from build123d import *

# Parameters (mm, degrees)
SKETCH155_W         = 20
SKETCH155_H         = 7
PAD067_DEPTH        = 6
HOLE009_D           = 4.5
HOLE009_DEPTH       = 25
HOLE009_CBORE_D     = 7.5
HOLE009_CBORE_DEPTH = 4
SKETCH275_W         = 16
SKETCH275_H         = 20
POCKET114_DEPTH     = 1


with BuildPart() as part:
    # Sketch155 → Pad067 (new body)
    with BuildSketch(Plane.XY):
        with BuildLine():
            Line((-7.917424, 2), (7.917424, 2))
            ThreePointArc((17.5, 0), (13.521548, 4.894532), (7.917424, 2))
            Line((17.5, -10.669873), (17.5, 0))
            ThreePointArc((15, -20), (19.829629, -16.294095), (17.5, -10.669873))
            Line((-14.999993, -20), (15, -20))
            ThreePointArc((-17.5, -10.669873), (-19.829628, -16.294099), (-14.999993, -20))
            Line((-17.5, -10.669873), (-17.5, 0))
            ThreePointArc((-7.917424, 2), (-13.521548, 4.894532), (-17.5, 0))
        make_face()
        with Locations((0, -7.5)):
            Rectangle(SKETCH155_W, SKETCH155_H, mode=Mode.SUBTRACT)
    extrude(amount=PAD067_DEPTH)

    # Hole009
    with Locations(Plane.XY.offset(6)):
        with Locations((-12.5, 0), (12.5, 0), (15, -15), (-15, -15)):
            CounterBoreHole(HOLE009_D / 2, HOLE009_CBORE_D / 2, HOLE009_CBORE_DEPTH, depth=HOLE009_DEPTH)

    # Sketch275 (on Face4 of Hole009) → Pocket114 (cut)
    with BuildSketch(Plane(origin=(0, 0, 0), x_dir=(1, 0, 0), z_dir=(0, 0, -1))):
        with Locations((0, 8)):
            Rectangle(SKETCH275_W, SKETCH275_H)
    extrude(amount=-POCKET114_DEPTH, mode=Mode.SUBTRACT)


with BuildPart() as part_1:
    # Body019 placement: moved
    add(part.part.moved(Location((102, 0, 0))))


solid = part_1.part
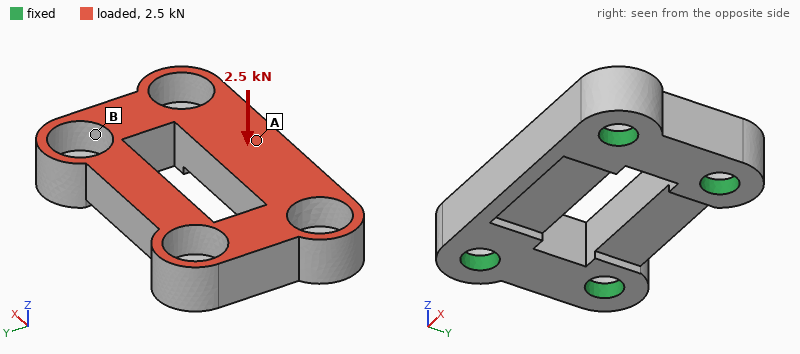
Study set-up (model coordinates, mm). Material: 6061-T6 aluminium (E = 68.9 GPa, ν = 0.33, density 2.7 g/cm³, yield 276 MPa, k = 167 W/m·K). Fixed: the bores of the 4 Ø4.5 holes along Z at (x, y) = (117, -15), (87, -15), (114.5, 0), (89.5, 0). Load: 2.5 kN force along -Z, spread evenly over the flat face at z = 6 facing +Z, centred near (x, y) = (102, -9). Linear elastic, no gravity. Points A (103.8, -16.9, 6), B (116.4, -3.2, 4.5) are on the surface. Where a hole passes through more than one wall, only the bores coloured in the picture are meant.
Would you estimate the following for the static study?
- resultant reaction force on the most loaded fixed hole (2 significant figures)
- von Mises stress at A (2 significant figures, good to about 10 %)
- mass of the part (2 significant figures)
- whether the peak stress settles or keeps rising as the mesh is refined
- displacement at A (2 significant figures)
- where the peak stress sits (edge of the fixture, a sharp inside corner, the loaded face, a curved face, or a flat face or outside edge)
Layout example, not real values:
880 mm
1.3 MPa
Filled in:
920 N
44 MPa
8.5 g
keeps rising
17 µm
edge of the fixture
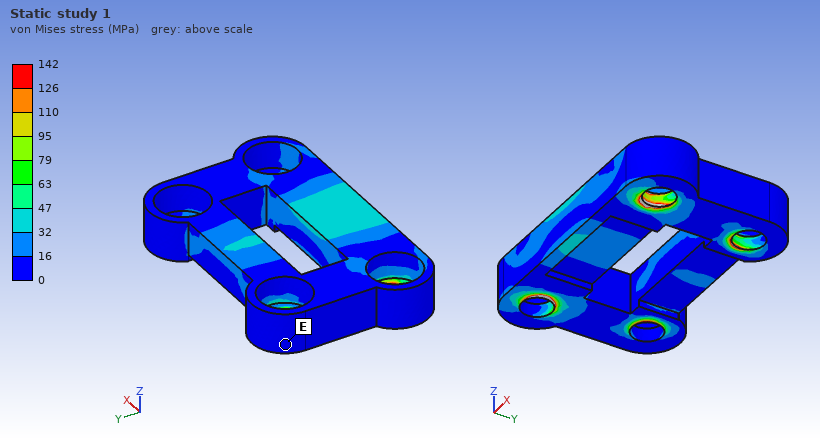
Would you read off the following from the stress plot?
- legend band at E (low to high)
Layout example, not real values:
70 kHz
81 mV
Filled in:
0 to 16 MPa
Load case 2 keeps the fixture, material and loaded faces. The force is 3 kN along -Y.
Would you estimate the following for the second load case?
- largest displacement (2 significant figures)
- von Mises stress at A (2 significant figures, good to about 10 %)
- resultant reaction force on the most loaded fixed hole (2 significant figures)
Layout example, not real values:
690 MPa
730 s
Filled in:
23 µm
16 MPa
900 N
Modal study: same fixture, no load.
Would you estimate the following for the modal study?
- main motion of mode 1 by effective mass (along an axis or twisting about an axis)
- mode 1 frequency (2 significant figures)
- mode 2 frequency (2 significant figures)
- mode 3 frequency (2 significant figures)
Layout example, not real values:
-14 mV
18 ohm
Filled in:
along Z
24 kHz
34 kHz
35 kHz
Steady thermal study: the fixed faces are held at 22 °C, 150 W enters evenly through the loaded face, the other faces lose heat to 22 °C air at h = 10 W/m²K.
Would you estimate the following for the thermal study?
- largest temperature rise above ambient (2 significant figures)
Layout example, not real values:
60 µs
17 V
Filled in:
48 K
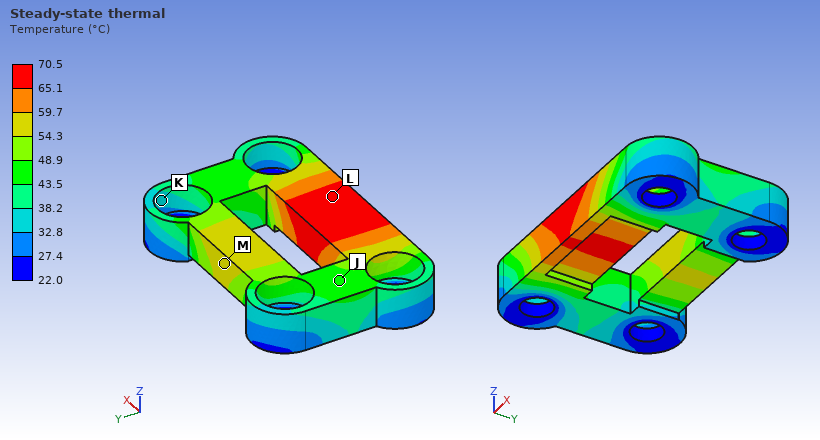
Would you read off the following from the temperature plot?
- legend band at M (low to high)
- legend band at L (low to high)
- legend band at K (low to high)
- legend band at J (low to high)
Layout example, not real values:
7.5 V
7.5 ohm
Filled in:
54.3 to 59.7 °C
65.1 to 70.5 °C
32.8 to 38.2 °C
43.5 to 48.9 °C
